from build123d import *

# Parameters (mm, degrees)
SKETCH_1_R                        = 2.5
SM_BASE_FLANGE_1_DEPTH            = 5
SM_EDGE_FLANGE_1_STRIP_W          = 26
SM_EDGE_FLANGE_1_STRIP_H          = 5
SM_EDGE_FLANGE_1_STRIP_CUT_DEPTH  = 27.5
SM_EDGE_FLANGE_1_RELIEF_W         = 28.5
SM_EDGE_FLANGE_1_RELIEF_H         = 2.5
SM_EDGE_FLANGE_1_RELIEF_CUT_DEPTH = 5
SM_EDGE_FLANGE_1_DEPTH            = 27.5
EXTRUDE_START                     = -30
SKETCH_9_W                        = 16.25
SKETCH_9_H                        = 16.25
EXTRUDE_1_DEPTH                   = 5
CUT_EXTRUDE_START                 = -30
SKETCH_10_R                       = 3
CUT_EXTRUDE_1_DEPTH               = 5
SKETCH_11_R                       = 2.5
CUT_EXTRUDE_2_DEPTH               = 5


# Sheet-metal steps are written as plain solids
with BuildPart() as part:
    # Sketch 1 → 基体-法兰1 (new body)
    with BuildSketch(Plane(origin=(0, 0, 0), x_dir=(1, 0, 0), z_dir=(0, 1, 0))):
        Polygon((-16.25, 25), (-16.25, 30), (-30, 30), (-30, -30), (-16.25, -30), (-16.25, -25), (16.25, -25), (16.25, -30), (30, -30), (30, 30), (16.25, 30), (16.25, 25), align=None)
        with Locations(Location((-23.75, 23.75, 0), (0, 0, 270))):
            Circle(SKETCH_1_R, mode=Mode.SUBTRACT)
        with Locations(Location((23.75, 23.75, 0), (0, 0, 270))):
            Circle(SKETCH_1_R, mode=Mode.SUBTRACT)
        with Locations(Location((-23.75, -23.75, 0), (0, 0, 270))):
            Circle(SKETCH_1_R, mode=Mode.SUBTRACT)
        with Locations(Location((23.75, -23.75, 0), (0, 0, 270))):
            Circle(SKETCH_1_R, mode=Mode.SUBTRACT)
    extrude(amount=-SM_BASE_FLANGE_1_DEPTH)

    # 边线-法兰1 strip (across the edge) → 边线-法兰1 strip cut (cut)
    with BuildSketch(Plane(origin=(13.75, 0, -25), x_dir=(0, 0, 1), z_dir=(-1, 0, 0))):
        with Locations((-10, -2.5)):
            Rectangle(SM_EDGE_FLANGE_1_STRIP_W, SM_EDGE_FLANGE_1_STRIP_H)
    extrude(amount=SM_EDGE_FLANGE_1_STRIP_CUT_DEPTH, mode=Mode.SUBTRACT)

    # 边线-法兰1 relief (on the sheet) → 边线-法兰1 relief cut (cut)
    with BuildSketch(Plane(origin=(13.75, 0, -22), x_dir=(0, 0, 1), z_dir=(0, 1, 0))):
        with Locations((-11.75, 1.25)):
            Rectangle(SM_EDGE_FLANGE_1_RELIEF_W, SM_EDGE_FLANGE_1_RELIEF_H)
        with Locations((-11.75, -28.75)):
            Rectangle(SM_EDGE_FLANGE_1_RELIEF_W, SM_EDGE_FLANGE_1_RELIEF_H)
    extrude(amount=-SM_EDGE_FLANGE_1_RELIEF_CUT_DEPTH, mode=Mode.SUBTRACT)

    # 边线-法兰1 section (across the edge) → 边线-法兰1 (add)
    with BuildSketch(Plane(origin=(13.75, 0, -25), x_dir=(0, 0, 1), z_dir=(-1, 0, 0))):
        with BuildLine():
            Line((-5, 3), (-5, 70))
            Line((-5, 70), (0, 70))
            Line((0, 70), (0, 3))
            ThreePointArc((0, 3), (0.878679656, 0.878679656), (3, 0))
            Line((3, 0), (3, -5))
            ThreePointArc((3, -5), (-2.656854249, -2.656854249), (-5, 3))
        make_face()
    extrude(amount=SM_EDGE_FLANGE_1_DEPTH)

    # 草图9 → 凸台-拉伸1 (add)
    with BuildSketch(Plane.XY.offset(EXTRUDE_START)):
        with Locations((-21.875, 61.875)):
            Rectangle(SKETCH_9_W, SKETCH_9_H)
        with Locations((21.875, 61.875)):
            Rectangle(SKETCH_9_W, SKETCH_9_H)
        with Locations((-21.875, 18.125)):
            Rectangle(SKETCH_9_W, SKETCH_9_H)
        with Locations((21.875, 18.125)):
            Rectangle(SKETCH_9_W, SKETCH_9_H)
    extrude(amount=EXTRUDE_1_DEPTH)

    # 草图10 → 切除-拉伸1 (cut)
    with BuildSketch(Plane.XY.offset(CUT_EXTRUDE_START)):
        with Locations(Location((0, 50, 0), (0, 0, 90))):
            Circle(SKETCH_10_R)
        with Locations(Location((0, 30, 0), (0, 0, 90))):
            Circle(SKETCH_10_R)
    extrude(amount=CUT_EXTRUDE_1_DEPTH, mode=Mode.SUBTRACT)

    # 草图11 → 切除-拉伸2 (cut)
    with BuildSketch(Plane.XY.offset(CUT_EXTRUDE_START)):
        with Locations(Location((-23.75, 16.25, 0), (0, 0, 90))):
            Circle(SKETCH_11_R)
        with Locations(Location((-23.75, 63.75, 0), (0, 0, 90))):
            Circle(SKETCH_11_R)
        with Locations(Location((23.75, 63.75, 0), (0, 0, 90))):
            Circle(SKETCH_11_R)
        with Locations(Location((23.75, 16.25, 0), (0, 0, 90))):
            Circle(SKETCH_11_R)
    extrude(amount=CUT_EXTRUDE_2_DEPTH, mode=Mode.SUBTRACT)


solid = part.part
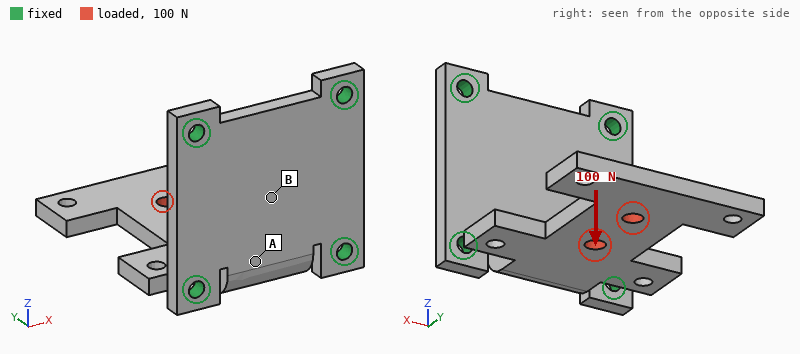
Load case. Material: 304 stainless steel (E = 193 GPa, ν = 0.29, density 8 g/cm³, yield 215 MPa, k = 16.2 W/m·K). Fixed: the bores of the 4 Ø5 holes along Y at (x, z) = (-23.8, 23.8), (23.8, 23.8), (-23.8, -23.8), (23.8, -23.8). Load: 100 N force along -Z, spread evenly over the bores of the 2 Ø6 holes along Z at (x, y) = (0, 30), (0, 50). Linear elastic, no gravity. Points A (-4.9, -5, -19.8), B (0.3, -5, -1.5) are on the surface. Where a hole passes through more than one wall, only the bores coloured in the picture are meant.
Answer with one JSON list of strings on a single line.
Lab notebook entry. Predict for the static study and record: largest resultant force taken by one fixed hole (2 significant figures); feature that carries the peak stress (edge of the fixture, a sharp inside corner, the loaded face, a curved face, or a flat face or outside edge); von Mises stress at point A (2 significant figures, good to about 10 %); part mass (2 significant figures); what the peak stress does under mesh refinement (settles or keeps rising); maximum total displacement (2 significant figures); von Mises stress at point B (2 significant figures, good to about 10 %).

["59 N", "a sharp inside corner", "27 MPa", "240 g", "keeps rising", "0.17 mm", "7.0 MPa"]
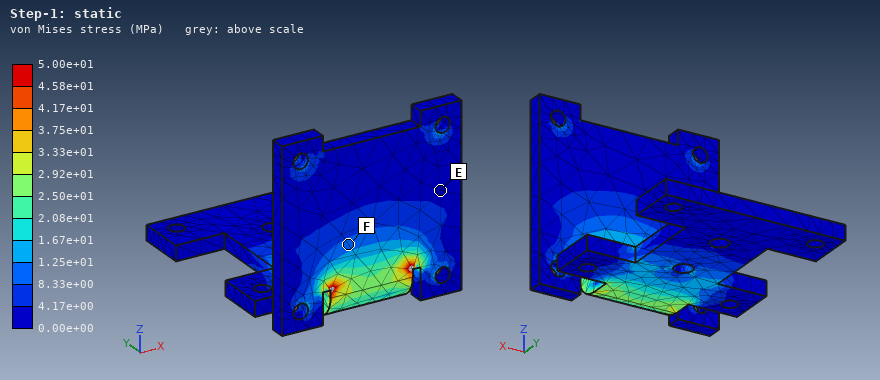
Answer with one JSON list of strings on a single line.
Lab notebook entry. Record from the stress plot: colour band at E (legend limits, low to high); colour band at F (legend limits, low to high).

["0.00e+00 to 4.17e+00 MPa", "8.33e+00 to 1.25e+01 MPa"]
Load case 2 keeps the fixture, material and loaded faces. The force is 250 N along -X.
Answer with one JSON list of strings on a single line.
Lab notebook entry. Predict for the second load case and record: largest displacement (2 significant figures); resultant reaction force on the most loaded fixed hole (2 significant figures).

["82 µm", "310 N"]
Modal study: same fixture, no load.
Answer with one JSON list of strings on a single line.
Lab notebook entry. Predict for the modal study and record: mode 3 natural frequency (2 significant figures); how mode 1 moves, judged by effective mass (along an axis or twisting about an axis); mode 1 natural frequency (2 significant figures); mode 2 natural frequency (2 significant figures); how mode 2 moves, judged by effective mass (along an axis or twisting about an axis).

["1600 Hz", "along Z", "440 Hz", "1000 Hz", "along X"]
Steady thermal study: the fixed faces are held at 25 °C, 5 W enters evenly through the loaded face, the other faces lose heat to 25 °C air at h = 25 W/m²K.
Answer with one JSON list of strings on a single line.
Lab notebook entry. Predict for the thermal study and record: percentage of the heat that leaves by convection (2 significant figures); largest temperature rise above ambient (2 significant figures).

["86 %", "35 K"]
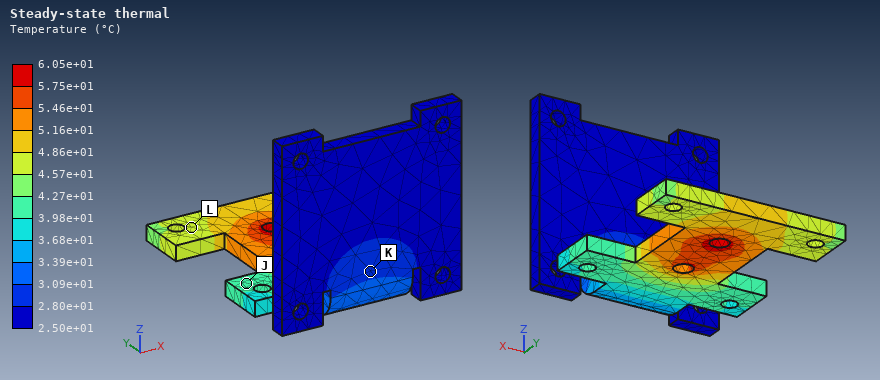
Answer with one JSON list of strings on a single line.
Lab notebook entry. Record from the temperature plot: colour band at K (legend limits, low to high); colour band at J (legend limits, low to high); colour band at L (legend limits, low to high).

["2.80e+01 to 3.09e+01 °C", "3.98e+01 to 4.27e+01 °C", "4.57e+01 to 4.86e+01 °C"]
